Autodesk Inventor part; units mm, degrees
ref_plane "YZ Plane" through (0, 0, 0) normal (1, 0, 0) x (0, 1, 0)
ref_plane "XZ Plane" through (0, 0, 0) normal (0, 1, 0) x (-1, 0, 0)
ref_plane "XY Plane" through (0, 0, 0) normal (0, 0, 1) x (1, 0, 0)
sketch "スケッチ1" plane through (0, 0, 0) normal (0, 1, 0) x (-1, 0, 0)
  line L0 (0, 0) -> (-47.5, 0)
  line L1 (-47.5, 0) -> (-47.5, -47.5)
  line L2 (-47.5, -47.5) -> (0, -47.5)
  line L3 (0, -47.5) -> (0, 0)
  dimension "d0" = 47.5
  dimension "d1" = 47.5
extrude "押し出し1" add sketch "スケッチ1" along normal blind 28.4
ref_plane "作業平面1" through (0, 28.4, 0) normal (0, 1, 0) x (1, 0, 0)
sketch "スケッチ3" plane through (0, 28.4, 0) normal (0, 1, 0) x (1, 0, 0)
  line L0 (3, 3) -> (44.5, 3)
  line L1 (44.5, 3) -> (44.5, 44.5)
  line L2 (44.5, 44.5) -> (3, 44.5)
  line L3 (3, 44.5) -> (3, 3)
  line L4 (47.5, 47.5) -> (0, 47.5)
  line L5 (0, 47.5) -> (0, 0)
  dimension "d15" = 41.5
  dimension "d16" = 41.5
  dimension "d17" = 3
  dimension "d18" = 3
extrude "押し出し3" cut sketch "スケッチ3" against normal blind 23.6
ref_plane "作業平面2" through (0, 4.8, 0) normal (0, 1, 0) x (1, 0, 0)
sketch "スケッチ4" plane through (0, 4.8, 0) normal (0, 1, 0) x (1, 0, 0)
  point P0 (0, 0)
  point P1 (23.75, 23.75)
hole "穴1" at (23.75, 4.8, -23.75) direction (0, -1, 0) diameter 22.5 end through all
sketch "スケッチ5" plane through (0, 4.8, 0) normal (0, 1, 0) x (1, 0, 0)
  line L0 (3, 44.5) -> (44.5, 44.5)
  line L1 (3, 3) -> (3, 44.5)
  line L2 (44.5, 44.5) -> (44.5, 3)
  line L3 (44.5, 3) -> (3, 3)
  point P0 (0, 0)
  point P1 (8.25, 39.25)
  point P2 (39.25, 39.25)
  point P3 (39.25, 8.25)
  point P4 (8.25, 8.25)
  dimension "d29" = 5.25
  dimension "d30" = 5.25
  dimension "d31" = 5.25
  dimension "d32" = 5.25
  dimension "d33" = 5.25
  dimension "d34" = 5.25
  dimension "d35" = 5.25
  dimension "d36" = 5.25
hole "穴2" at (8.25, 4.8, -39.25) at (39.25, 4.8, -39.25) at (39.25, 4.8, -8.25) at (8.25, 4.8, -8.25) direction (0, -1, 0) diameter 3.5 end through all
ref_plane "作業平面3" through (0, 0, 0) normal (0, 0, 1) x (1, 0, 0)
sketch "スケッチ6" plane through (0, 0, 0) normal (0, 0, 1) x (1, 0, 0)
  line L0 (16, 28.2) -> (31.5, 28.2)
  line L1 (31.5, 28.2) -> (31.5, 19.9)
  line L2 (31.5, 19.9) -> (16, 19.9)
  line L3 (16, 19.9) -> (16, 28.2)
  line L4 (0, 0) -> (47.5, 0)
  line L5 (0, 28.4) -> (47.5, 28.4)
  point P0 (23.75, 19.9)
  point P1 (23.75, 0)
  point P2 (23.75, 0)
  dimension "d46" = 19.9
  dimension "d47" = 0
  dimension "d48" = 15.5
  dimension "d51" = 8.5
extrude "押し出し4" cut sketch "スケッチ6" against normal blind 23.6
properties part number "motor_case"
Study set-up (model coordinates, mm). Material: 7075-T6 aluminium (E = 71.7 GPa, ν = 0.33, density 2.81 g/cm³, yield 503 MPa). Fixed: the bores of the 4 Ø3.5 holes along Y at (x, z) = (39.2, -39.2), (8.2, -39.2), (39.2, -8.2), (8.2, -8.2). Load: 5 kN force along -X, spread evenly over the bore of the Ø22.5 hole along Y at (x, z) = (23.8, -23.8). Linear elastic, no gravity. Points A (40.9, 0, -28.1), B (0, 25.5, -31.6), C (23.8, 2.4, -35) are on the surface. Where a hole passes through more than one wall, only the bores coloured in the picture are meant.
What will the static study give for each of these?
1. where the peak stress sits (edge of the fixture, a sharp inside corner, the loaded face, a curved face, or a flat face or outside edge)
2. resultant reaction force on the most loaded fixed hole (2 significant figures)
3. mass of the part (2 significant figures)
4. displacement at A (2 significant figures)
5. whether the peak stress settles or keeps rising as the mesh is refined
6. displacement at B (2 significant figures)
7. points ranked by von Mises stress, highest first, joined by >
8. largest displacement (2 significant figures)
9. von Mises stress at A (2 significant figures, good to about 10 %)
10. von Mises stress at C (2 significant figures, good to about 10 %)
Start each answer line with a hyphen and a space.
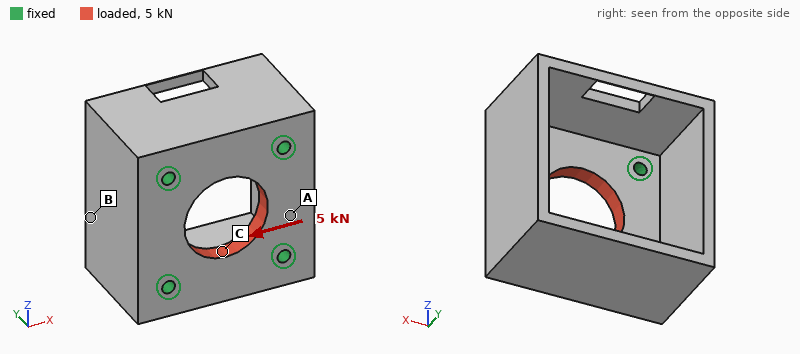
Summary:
- edge of the fixture
- 1.3 kN
- 59 g
- 5.3 µm
- keeps rising
- 2.4 µm
- C > A > B
- 6.9 µm
- 13 MPa
- 25 MPa
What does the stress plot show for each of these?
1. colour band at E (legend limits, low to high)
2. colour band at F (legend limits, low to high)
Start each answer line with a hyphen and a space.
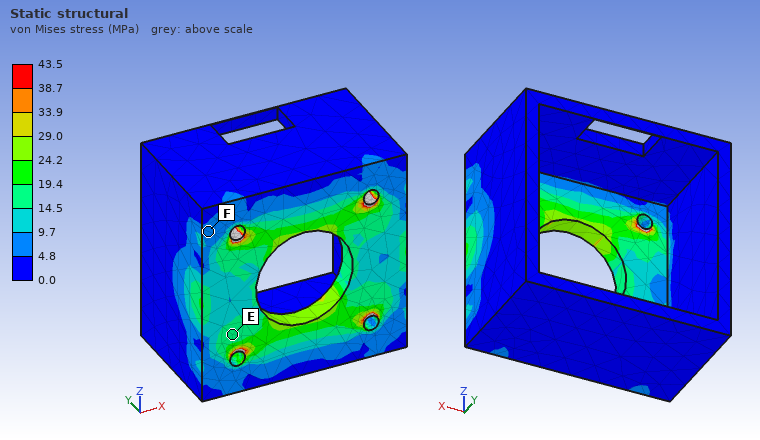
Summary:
- 14.5 to 19.4 MPa
- 4.8 to 9.7 MPa
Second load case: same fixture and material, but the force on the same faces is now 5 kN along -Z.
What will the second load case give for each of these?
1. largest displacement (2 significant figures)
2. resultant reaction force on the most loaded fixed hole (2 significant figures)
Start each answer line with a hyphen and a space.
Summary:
- 7.0 µm
- 1.3 kN
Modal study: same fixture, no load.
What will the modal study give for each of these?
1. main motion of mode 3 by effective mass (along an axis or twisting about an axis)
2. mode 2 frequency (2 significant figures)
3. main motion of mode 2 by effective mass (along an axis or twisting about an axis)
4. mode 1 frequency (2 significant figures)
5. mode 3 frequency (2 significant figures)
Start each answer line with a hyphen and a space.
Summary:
- along Z
- 7600 Hz
- along X
- 6700 Hz
- 8400 Hz
